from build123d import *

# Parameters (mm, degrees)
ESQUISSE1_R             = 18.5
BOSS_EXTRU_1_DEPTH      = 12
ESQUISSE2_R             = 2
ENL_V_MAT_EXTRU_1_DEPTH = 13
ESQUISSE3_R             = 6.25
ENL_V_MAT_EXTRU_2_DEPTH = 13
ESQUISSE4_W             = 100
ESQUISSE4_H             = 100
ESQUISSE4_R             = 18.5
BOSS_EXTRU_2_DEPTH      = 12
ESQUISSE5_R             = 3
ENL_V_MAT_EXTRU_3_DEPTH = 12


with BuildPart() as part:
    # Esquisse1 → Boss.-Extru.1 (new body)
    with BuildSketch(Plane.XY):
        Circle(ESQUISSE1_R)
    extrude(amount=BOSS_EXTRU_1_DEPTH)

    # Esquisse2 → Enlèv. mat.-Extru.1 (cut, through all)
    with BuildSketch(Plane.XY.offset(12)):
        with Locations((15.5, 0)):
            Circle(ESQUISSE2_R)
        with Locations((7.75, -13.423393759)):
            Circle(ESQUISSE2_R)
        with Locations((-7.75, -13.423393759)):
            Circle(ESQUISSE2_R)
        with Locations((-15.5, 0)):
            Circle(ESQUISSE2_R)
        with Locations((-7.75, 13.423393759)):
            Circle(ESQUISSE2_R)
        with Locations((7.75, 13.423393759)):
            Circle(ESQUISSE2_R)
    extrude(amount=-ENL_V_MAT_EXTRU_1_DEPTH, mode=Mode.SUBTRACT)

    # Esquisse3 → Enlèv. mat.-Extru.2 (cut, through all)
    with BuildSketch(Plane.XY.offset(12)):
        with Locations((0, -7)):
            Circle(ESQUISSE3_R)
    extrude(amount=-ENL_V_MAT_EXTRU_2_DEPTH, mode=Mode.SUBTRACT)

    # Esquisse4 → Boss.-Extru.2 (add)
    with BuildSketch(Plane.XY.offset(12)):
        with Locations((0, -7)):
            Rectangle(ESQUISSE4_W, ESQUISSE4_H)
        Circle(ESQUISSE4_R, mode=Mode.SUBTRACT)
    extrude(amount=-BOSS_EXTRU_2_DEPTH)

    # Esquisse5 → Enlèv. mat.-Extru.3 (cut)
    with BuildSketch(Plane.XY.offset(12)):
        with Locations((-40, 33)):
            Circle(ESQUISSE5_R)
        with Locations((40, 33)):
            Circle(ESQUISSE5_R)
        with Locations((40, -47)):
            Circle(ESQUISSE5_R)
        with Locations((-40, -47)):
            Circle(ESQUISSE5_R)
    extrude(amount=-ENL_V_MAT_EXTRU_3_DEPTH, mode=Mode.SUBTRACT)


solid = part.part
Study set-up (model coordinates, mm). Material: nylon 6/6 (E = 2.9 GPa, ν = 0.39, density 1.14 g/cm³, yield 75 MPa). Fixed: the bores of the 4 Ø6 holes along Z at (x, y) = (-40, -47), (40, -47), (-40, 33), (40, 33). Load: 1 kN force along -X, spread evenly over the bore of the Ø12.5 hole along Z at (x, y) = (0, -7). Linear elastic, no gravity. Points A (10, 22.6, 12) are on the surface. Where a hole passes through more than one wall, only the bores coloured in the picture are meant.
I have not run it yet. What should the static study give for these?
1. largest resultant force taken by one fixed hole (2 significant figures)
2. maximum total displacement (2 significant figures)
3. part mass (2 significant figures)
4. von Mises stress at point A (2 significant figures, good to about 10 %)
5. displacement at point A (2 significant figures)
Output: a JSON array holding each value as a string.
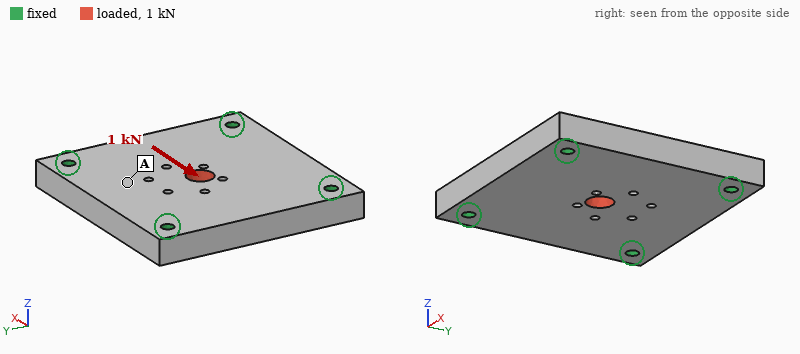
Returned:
["290 N", "30 µm", "130 g", "0.64 MPa", "8.7 µm"]
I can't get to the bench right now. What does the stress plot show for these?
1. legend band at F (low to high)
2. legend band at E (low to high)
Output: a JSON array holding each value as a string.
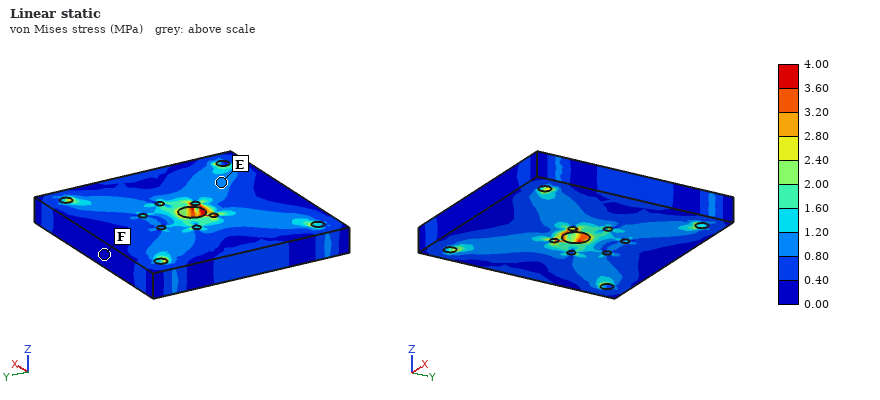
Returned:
["0.00 to 0.40 MPa", "0.80 to 1.20 MPa"]
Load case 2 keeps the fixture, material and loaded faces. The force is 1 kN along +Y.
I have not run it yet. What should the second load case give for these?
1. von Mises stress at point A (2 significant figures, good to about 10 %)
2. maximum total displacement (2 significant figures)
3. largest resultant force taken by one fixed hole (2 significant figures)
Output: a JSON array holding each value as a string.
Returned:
["0.61 MPa", "29 µm", "280 N"]
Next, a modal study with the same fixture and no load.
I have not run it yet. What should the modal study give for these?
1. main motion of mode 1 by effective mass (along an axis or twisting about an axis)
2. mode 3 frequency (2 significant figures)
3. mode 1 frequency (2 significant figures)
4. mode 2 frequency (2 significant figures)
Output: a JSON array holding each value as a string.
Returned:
["along Z", "2900 Hz", "1800 Hz", "2900 Hz"]
